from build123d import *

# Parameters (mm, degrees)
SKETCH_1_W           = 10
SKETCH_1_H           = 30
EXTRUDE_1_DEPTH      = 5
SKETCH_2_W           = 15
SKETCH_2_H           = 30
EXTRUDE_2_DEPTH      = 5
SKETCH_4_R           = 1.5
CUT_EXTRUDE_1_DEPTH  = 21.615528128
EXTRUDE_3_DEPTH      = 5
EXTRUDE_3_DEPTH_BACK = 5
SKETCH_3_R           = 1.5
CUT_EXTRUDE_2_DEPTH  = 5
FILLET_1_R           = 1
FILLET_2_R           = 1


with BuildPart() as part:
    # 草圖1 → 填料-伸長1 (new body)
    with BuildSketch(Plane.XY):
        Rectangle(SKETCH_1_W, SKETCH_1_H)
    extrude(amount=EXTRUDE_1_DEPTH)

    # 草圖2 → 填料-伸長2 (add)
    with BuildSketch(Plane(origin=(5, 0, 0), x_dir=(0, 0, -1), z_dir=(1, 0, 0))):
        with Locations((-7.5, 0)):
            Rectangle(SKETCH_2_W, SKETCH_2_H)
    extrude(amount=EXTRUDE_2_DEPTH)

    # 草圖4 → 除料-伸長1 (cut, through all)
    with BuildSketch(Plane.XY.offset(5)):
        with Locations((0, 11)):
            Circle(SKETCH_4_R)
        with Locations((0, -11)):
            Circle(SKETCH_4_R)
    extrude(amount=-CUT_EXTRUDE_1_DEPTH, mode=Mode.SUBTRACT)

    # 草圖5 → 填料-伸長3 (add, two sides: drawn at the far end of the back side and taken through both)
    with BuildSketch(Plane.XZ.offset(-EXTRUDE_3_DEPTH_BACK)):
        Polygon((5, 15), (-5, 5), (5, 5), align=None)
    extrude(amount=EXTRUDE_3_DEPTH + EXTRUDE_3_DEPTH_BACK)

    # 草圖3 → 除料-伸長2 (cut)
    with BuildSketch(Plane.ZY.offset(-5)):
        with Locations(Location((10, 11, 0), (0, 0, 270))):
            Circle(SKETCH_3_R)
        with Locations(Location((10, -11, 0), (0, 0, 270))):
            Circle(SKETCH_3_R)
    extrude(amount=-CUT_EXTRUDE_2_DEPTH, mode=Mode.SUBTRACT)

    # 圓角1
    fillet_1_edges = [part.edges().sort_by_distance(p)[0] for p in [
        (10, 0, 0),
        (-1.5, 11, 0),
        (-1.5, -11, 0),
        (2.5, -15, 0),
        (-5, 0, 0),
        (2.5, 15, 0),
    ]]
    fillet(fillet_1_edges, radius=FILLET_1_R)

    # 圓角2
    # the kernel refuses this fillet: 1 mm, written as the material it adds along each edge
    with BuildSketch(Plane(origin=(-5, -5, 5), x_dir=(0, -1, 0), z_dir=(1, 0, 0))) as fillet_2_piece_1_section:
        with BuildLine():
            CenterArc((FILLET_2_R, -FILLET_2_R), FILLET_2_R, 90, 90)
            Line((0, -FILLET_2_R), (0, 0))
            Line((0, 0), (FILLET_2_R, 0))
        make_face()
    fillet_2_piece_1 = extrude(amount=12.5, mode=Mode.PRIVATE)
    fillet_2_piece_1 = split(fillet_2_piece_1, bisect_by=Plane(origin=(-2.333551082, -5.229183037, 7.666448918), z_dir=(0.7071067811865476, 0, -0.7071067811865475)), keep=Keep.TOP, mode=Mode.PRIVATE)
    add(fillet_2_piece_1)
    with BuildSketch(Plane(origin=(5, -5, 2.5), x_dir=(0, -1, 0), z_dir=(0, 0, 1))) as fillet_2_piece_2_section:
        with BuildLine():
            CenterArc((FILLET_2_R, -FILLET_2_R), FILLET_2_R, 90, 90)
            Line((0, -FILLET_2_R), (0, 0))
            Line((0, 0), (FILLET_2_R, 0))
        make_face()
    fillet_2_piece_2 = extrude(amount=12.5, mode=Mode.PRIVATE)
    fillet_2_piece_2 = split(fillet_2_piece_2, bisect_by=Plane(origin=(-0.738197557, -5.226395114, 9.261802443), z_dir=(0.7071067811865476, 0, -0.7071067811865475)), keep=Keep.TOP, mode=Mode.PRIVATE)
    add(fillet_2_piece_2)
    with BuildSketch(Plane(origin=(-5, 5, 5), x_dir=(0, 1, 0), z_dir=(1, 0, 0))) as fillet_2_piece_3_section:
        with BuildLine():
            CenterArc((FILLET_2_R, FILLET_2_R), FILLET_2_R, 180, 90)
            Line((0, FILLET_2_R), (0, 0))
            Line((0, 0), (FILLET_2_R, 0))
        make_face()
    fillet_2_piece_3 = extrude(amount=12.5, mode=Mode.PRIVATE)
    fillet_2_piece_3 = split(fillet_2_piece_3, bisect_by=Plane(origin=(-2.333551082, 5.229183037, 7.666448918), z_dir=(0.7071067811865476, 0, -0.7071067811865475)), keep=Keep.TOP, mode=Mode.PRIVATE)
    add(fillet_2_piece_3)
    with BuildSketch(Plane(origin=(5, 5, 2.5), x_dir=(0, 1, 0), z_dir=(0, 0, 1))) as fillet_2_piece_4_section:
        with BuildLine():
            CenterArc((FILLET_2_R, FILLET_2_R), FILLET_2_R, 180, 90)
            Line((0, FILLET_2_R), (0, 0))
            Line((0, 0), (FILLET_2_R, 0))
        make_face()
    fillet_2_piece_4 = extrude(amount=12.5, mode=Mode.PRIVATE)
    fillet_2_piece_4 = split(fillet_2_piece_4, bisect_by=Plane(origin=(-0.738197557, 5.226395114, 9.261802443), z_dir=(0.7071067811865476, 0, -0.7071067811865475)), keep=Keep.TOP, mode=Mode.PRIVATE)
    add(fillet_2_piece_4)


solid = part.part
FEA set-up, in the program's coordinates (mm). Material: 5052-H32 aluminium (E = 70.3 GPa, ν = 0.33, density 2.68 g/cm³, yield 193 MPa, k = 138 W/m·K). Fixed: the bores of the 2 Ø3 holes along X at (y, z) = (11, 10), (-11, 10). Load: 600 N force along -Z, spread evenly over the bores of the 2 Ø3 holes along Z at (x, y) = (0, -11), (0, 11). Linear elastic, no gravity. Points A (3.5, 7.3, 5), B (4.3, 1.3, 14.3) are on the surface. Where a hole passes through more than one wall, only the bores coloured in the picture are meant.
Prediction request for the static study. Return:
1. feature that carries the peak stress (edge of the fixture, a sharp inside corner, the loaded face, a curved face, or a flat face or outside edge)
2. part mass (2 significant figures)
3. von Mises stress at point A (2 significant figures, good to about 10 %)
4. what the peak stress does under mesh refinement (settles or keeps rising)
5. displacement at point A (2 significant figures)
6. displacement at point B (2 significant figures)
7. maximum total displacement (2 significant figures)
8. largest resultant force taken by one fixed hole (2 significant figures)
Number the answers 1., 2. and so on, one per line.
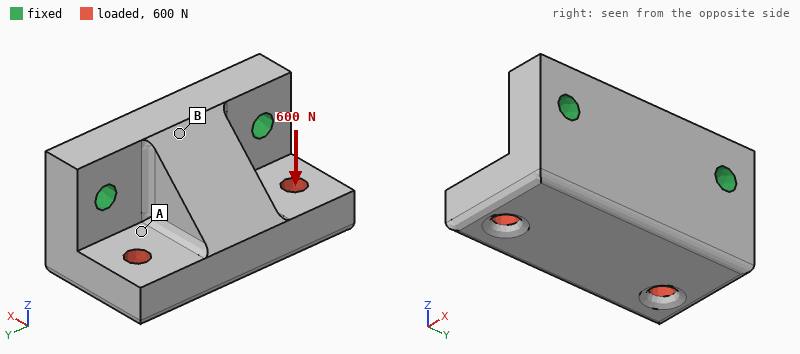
1. edge of the fixture
2. 11 g
3. 14 MPa
4. keeps rising
5. 6.4 µm
6. 6.2 µm
7. 22 µm
8. 300 N
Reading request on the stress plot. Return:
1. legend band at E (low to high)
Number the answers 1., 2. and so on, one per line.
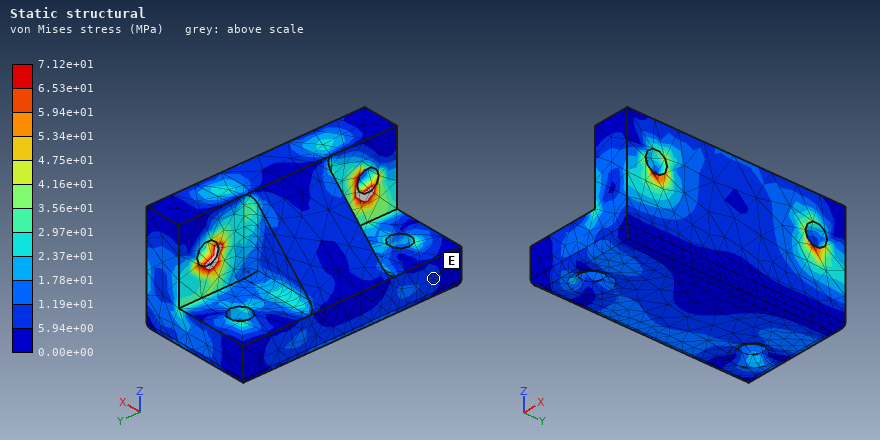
1. 5.94e+00 to 1.19e+01 MPa
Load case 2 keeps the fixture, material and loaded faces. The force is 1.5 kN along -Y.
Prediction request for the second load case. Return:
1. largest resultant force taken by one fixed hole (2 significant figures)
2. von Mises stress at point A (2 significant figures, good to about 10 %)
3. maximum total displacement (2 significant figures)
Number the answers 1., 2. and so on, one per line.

1. 1.0 kN
2. 29 MPa
3. 12 µm
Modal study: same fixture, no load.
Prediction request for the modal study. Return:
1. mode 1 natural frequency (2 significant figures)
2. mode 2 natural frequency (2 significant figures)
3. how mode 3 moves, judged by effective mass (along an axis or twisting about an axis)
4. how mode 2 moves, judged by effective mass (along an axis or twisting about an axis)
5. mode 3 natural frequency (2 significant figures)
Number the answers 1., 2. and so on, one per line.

1. 13 kHz
2. 27 kHz
3. along X
4. along Y
5. 32 kHz
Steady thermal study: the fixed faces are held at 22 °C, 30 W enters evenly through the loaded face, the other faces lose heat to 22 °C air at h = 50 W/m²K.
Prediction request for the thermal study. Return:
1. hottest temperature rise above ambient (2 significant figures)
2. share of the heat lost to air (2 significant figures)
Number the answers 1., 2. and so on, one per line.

1. 25 K
2. 3.5 %
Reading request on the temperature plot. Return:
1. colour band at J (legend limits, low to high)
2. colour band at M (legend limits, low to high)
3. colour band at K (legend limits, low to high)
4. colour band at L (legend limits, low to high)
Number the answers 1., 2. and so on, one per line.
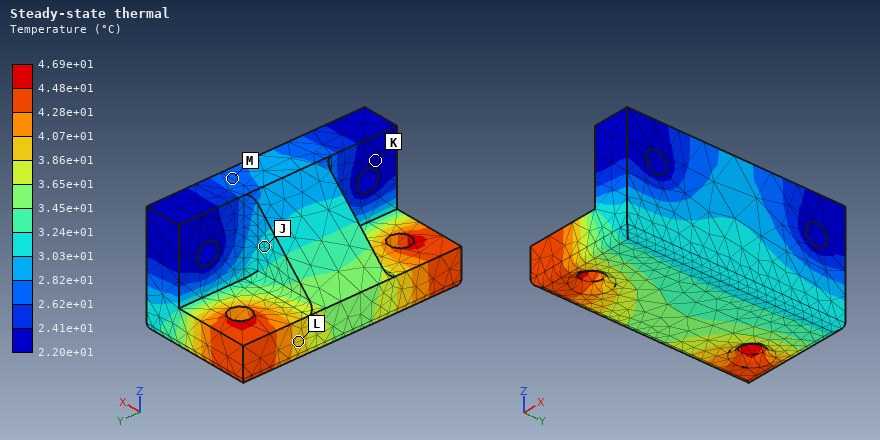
1. 3.03e+01 to 3.24e+01 °C
2. 2.62e+01 to 2.82e+01 °C
3. 2.20e+01 to 2.41e+01 °C
4. 3.86e+01 to 4.07e+01 °C
